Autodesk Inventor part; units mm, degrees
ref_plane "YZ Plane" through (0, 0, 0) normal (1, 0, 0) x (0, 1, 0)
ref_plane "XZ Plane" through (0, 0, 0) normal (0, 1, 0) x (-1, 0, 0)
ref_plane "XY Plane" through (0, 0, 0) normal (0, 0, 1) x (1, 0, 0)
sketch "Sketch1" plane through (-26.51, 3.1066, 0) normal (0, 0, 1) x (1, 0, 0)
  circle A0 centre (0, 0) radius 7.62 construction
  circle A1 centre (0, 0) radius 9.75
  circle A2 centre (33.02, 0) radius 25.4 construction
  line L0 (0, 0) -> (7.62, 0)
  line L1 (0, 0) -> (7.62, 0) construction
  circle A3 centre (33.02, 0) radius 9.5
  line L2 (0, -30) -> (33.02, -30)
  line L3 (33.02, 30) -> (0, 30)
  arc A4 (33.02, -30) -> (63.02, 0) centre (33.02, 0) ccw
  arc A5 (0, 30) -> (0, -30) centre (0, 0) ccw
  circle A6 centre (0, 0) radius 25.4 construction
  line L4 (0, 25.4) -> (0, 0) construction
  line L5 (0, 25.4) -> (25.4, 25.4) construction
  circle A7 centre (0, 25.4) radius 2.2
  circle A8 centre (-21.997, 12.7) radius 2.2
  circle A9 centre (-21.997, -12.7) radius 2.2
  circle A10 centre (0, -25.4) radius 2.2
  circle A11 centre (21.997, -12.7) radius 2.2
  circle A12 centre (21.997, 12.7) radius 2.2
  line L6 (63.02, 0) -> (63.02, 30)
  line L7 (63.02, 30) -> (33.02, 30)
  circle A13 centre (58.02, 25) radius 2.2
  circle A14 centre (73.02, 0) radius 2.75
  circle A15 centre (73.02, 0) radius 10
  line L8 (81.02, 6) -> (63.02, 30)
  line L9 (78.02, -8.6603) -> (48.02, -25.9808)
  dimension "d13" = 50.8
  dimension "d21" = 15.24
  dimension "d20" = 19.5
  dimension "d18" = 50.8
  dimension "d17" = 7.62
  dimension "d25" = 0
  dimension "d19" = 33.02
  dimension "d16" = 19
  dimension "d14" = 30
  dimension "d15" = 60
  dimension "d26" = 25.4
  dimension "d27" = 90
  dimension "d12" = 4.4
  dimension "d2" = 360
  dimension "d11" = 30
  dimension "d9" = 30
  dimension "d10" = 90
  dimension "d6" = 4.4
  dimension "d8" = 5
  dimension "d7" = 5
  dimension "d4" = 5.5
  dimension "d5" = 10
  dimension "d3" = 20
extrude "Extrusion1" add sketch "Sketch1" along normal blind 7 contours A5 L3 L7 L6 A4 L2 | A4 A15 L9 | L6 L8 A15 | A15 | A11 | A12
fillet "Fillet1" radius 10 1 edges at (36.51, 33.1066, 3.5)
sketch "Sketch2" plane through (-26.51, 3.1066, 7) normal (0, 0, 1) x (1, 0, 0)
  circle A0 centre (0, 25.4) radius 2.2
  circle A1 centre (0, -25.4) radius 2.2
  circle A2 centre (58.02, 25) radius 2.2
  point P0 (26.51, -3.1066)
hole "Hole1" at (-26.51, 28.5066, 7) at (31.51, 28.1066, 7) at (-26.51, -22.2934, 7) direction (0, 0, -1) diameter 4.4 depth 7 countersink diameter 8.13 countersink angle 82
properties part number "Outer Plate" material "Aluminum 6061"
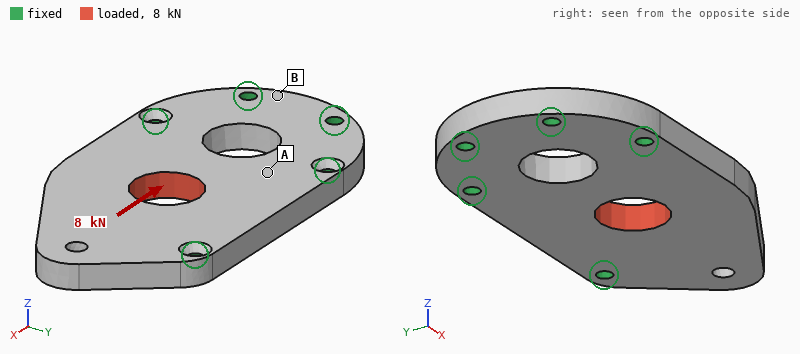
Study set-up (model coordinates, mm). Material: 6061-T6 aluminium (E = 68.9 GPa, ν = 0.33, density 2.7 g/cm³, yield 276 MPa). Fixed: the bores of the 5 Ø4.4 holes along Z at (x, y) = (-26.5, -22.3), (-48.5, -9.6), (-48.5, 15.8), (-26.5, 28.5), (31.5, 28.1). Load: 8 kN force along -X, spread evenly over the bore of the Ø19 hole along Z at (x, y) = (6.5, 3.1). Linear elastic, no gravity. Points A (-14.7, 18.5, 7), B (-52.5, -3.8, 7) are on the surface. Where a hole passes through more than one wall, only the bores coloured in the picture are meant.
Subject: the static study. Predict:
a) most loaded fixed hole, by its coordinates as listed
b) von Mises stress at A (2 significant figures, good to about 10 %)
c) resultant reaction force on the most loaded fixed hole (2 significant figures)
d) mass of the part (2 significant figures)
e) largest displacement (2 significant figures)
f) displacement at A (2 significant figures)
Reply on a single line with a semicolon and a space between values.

(-26.5, -22.3); 16 MPa; 2.6 kN; 93 g; 17 µm; 5.4 µm
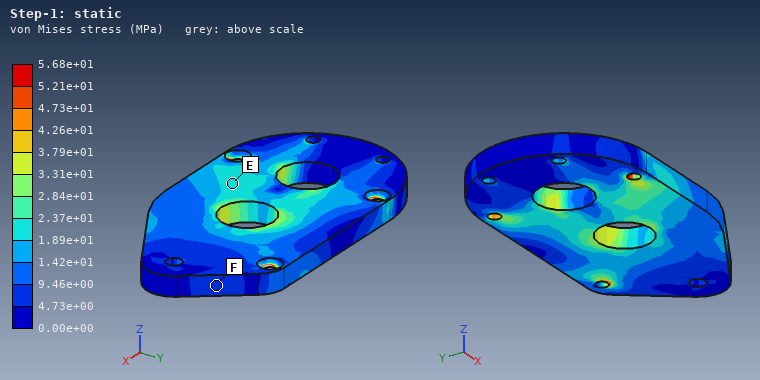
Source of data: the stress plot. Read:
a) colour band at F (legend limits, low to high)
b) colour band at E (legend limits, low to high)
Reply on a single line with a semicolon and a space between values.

4.73e+00 to 9.46e+00 MPa; 1.89e+01 to 2.37e+01 MPa
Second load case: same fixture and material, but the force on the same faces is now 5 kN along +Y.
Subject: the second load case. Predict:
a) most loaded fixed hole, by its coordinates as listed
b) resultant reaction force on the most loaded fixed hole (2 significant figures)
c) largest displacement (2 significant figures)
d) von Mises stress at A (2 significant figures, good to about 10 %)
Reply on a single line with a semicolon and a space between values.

(31.5, 28.1); 2.6 kN; 13 µm; 13 MPa
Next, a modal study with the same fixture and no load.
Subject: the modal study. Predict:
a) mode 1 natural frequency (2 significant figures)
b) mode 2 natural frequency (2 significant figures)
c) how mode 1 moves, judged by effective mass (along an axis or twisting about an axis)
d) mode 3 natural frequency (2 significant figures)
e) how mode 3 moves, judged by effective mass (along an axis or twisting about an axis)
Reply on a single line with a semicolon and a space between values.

2800 Hz; 5800 Hz; along Z; 8700 Hz; along Z
